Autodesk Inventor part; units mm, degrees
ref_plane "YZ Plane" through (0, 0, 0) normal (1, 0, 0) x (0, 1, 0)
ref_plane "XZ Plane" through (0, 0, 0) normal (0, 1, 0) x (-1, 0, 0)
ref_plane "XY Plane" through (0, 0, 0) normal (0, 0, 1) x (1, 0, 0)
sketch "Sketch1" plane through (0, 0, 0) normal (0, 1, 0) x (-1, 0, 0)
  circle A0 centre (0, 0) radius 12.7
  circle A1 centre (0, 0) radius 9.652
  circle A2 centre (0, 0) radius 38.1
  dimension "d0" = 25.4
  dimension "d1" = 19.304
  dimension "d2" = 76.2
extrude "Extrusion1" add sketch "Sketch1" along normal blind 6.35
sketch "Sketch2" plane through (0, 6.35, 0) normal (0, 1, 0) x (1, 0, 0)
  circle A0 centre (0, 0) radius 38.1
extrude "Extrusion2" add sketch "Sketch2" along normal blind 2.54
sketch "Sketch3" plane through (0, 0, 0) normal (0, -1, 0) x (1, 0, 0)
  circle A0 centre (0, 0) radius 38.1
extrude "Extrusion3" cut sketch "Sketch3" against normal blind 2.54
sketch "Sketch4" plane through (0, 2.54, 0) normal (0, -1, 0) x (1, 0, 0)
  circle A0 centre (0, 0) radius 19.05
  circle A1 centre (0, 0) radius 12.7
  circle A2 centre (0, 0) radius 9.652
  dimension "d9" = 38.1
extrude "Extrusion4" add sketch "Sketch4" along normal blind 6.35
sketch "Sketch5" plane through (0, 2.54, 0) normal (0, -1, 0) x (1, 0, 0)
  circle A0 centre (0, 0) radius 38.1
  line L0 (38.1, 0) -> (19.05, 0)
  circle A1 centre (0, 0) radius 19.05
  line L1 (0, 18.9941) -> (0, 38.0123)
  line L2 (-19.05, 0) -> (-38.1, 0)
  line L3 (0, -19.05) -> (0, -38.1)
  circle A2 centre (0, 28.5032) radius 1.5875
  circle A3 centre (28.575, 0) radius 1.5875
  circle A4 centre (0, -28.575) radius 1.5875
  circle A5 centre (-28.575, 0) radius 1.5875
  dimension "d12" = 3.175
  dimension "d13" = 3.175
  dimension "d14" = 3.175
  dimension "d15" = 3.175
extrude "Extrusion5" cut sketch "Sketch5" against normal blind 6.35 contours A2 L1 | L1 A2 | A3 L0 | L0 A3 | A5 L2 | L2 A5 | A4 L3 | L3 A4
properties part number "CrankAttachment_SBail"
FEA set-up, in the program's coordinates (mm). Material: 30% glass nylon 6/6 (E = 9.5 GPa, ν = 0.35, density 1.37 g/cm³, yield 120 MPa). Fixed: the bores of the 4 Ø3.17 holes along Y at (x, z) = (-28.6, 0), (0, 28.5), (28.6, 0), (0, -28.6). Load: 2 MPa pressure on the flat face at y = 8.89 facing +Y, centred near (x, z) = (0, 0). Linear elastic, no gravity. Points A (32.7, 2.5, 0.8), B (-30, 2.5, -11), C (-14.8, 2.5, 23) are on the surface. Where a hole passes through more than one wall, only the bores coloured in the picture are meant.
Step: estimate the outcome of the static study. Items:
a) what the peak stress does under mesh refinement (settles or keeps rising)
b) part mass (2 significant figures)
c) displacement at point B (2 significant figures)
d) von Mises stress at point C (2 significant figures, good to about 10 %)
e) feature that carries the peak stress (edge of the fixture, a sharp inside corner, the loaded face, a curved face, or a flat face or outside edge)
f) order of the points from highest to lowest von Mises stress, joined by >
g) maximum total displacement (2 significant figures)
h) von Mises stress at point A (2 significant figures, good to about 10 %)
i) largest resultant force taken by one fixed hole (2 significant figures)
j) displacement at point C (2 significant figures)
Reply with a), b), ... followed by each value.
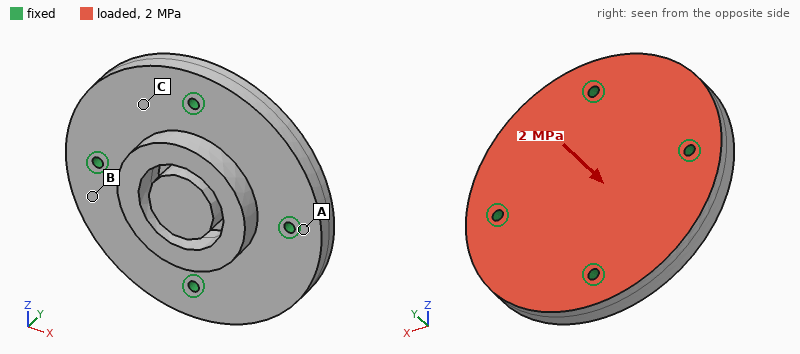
a) keeps rising
b) 46 g
c) 0.087 mm
d) 20 MPa
e) edge of the fixture
f) A > C > B
g) 0.20 mm
h) 41 MPa
i) 2.3 kN
j) 0.12 mm
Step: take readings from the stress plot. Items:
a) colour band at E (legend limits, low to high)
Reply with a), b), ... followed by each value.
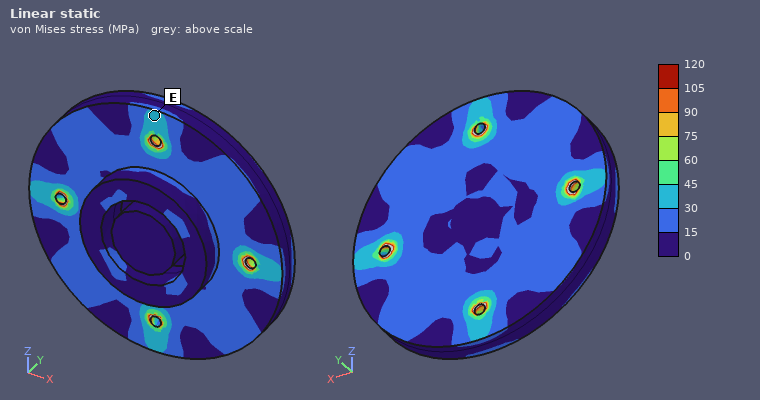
a) 30 to 45 MPa
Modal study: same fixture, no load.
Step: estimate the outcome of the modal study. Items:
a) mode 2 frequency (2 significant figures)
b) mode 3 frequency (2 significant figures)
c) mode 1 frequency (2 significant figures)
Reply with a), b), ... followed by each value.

a) 6100 Hz
b) 6200 Hz
c) 5600 Hz
